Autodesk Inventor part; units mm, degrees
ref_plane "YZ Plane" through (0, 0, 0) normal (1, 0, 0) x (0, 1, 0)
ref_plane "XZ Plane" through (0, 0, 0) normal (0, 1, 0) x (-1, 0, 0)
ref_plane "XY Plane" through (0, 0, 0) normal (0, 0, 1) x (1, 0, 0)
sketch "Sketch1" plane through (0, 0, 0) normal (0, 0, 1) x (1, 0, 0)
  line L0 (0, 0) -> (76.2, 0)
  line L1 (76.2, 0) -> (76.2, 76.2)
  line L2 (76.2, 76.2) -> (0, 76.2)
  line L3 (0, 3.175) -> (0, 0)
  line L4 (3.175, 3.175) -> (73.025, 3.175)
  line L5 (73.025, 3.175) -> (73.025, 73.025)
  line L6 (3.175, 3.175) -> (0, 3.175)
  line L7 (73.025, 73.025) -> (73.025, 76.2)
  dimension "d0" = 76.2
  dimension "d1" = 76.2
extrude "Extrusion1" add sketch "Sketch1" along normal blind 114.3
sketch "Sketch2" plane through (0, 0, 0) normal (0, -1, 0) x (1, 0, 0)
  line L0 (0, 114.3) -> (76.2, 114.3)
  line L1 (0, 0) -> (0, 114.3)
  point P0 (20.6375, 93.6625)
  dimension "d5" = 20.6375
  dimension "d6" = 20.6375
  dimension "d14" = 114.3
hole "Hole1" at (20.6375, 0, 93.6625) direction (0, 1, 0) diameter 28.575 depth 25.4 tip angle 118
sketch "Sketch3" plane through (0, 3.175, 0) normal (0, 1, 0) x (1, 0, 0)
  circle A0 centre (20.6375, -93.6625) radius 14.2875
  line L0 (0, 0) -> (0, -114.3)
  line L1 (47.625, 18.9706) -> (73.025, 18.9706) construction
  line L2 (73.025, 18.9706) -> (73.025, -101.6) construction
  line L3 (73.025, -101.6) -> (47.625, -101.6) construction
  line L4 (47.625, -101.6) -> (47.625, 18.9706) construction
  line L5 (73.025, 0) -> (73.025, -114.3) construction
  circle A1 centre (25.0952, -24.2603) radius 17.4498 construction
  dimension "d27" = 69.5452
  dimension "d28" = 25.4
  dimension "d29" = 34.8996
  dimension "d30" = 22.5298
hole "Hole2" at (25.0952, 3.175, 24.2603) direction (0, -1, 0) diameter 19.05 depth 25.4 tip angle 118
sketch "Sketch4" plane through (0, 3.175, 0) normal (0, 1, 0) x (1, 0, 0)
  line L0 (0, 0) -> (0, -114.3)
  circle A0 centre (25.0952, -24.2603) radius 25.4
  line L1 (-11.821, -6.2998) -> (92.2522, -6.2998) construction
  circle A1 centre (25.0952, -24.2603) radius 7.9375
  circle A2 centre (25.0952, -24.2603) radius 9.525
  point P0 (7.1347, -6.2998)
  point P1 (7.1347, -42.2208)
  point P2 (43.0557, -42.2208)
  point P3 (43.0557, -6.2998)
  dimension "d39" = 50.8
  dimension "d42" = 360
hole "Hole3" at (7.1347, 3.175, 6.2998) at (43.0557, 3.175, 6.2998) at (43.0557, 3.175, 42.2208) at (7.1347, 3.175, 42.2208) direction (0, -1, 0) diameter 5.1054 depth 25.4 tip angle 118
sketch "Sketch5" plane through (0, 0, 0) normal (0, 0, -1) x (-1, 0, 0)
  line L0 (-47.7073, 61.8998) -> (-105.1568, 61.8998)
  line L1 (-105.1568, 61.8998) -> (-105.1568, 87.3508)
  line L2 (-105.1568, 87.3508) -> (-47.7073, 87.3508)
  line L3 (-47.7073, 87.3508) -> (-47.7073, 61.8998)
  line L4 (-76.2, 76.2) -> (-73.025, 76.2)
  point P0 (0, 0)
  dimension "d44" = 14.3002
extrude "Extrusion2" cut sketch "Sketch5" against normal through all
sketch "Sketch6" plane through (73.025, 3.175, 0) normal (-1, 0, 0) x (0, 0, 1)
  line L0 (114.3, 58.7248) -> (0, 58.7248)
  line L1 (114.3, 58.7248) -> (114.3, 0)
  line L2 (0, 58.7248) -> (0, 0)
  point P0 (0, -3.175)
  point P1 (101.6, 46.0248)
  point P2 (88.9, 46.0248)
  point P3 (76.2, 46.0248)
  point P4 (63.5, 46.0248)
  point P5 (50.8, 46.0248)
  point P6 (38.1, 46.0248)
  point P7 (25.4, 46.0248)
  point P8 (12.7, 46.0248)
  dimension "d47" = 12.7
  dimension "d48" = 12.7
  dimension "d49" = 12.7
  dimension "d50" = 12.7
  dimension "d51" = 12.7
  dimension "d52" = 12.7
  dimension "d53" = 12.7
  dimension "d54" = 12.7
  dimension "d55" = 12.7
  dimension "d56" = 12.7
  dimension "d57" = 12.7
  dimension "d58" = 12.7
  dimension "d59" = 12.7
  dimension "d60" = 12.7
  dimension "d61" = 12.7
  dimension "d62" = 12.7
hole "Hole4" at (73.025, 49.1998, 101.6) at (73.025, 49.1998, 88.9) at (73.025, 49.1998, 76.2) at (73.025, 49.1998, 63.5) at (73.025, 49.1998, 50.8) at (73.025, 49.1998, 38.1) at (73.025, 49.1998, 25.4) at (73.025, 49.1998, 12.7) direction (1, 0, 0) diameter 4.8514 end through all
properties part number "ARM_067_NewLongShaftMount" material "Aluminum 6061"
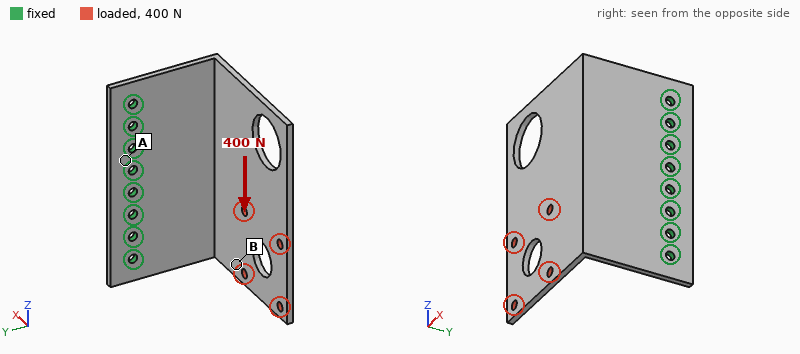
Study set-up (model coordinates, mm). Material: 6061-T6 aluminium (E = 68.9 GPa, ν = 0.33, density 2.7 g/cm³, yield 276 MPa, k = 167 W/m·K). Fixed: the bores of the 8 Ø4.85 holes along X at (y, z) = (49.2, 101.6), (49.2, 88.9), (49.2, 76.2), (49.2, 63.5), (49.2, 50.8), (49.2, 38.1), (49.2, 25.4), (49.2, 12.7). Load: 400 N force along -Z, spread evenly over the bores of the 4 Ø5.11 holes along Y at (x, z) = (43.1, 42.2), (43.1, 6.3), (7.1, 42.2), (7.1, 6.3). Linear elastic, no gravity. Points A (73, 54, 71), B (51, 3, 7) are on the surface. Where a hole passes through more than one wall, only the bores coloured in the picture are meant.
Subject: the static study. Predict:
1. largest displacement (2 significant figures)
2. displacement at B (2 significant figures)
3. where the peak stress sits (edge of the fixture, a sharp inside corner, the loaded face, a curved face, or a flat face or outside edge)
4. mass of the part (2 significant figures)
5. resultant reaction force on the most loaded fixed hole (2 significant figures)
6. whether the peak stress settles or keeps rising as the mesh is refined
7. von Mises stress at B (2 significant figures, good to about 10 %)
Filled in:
0.97 mm
0.55 mm
edge of the fixture
120 g
240 N
keeps rising
22 MPa
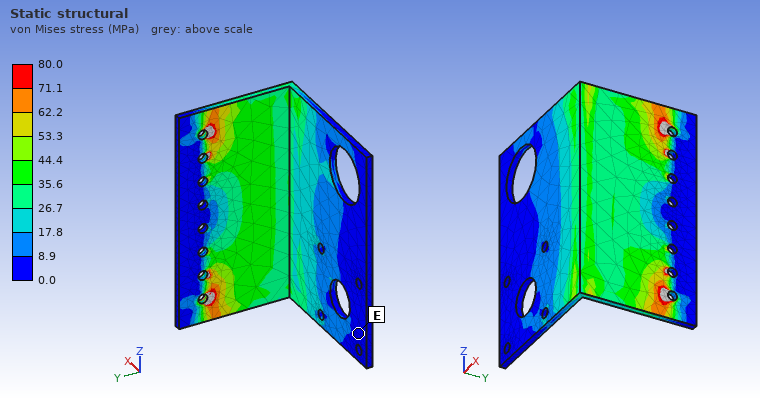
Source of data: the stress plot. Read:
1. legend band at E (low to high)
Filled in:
0.0 to 8.9 MPa
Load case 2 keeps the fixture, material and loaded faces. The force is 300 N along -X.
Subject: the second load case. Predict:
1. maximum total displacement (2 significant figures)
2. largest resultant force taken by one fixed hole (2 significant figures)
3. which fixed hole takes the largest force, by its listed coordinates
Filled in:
1.5 mm
110 N
(49.2, 12.7)
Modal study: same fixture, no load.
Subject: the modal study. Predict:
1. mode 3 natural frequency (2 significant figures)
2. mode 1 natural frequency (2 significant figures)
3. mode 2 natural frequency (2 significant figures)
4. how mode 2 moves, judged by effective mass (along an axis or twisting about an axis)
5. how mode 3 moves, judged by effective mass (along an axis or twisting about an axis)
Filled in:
760 Hz
260 Hz
490 Hz
along Z
along X
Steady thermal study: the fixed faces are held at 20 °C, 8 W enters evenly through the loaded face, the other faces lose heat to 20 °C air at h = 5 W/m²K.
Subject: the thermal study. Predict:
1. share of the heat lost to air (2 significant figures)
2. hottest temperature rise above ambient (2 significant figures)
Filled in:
12 %
18 K
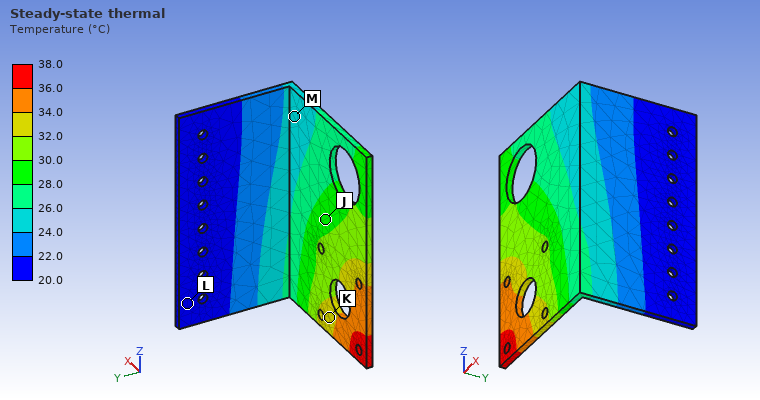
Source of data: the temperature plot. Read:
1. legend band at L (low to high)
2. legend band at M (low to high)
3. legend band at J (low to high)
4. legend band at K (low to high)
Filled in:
20.0 to 22.0 °C
24.0 to 26.0 °C
28.0 to 30.0 °C
32.0 to 34.0 °C
